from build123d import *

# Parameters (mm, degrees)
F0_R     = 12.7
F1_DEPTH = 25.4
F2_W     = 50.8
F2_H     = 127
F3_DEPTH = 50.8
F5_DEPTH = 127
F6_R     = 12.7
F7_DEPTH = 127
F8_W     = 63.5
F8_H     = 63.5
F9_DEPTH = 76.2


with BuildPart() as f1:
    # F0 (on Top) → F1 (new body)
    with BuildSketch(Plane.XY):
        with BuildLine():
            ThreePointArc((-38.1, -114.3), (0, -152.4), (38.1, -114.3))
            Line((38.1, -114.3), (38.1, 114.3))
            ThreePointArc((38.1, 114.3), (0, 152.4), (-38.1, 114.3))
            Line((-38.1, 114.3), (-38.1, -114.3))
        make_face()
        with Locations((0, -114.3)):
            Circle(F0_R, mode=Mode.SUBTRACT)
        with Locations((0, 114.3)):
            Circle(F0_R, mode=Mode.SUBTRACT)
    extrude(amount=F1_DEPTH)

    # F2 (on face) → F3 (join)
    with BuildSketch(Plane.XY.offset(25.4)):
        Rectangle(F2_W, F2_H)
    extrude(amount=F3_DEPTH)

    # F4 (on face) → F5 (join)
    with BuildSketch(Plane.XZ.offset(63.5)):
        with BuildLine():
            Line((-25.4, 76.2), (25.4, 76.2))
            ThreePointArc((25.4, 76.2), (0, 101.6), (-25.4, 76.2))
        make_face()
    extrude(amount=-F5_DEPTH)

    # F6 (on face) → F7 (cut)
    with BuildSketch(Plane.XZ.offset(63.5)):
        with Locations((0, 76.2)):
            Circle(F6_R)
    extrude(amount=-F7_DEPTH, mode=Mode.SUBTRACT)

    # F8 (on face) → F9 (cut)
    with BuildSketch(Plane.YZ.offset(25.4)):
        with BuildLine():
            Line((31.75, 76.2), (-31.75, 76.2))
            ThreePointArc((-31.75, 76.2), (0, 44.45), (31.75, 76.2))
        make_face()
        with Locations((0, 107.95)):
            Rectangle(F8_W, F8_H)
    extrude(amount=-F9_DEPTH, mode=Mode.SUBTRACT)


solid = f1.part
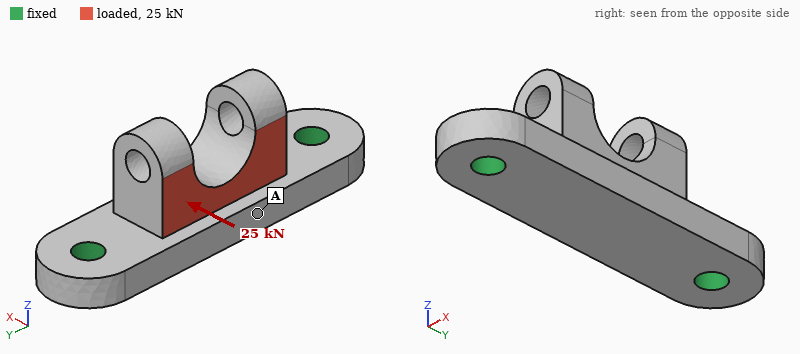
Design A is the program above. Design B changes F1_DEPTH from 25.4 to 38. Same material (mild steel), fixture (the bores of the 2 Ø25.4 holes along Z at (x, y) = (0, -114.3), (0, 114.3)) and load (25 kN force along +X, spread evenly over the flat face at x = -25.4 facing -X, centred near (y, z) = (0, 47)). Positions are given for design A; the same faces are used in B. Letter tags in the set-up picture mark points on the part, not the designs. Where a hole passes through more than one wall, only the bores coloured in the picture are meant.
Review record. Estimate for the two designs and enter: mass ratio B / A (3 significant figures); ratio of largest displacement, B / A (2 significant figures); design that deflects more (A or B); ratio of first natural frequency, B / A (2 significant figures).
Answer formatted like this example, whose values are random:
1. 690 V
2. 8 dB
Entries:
1. 1.23
2. 0.46
3. A
4. 1.5
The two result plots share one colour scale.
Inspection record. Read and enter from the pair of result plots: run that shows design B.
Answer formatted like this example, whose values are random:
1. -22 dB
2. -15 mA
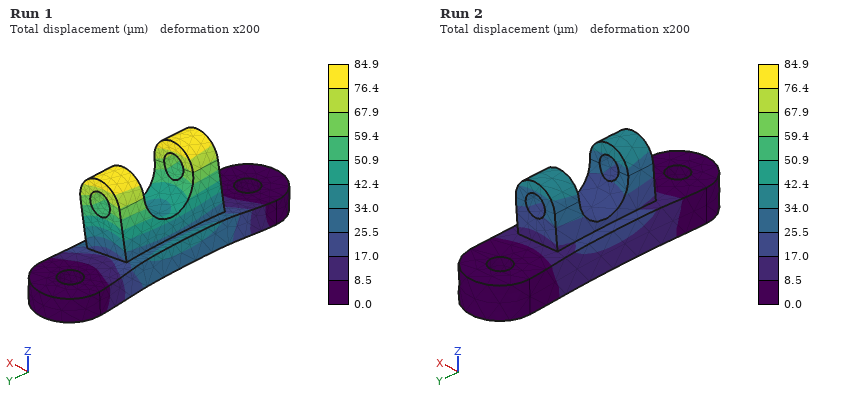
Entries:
1. Run 2
